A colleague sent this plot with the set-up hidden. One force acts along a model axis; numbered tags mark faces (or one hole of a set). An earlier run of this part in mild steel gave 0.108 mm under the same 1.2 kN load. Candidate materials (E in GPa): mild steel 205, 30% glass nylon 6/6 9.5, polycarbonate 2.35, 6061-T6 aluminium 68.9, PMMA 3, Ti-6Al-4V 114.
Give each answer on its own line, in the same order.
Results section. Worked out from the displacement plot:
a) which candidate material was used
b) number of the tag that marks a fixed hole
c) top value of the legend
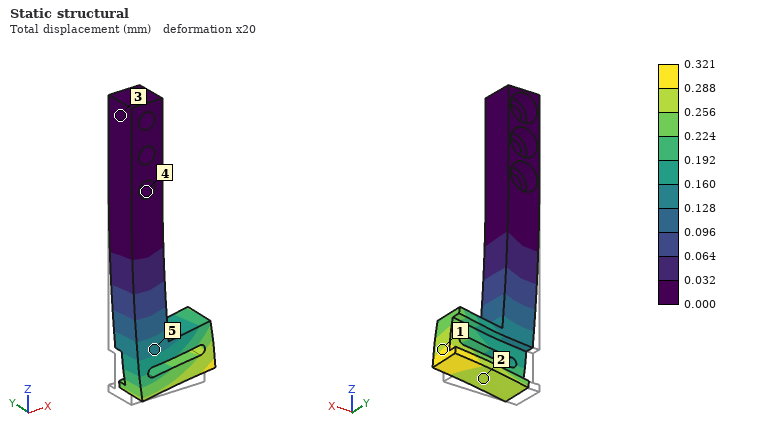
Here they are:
6061-T6 aluminium
4
0.321 mm
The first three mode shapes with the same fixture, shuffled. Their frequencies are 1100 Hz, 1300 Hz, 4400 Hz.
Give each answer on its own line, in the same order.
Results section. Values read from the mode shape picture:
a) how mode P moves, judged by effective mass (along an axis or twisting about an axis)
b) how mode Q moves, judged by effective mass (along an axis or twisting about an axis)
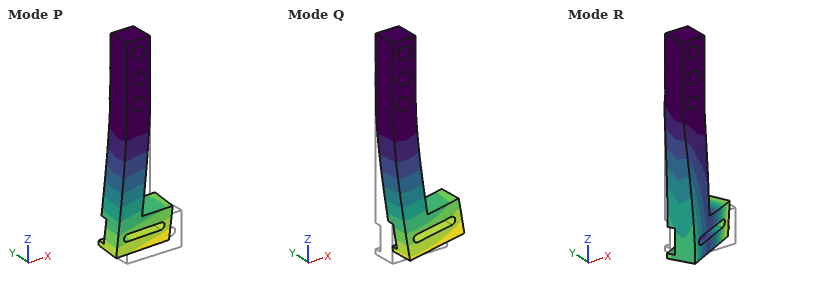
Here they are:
along Y
along X
